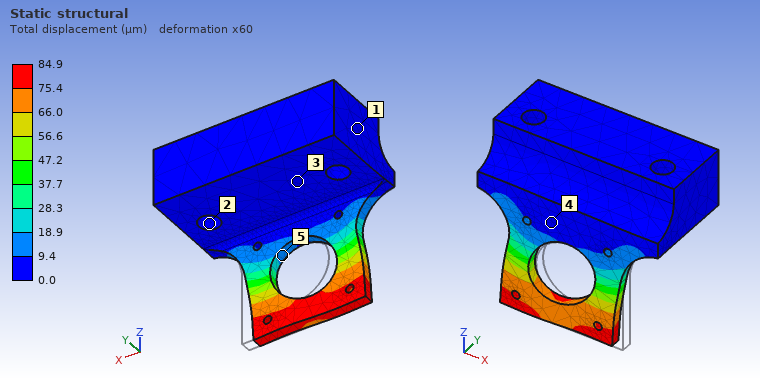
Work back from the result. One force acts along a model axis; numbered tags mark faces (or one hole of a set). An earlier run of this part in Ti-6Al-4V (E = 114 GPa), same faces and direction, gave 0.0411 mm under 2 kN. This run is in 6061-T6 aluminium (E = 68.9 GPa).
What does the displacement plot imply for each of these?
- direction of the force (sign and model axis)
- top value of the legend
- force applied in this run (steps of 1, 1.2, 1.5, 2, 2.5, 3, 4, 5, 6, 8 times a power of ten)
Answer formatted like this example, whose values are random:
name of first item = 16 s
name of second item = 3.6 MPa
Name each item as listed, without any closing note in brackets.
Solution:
direction of the force = -X
top value of the legend = 84.9 µm
force applied in this run = 2.5 kN
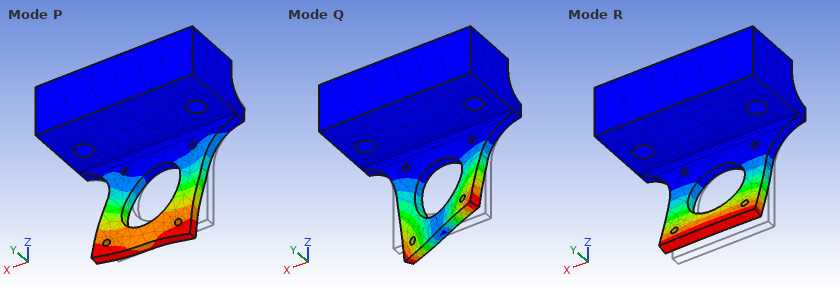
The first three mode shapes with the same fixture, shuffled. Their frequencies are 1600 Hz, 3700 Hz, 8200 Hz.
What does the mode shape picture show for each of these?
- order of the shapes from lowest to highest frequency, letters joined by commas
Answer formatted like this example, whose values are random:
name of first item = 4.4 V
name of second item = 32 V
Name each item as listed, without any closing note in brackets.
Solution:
order of the shapes from lowest to highest frequency, letters joined by commas = R, Q, P
